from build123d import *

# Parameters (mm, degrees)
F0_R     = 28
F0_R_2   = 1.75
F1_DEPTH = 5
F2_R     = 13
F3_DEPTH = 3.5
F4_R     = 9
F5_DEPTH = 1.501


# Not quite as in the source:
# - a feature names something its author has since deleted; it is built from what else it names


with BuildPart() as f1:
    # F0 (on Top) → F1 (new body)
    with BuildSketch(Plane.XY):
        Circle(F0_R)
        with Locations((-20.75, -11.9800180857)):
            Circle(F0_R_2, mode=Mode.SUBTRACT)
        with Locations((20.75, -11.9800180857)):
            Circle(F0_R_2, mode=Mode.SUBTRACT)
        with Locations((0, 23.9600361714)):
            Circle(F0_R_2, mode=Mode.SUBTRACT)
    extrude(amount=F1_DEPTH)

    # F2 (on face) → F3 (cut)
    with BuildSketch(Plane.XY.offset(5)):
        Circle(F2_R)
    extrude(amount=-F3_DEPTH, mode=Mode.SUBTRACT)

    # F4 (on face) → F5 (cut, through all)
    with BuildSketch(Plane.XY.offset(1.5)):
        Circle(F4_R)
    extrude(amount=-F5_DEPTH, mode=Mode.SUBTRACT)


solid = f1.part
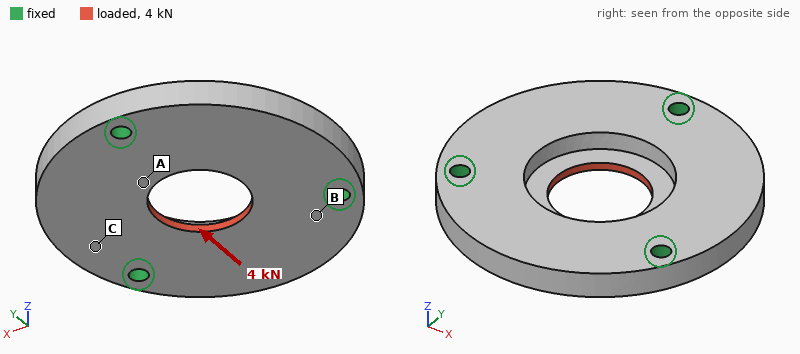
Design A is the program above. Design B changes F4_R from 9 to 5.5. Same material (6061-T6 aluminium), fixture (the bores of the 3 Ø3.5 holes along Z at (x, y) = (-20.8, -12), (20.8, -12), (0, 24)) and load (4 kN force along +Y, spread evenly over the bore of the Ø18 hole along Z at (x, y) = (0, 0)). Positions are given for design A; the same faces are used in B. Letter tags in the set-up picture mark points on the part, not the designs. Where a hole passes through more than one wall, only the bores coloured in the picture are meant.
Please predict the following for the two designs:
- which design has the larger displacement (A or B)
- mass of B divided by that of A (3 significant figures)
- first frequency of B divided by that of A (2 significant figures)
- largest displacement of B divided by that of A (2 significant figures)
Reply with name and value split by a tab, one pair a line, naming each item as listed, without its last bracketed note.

which design has the larger displacement	B
mass of B divided by that of A	1.02
first frequency of B divided by that of A	1.0
largest displacement of B divided by that of A	1.1
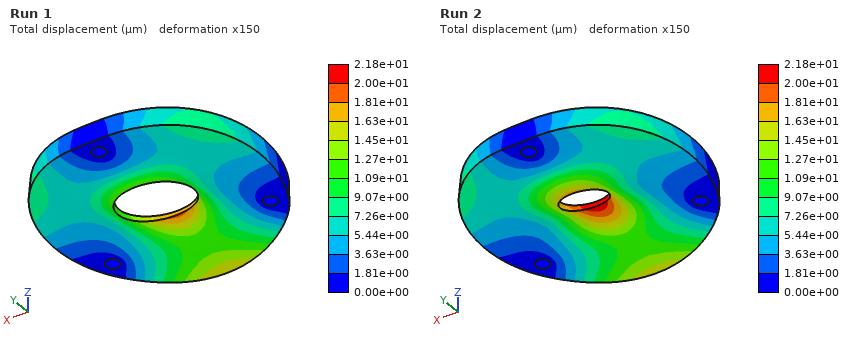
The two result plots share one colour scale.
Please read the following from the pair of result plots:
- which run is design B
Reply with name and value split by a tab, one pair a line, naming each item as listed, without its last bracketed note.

which run is design B	Run 2
